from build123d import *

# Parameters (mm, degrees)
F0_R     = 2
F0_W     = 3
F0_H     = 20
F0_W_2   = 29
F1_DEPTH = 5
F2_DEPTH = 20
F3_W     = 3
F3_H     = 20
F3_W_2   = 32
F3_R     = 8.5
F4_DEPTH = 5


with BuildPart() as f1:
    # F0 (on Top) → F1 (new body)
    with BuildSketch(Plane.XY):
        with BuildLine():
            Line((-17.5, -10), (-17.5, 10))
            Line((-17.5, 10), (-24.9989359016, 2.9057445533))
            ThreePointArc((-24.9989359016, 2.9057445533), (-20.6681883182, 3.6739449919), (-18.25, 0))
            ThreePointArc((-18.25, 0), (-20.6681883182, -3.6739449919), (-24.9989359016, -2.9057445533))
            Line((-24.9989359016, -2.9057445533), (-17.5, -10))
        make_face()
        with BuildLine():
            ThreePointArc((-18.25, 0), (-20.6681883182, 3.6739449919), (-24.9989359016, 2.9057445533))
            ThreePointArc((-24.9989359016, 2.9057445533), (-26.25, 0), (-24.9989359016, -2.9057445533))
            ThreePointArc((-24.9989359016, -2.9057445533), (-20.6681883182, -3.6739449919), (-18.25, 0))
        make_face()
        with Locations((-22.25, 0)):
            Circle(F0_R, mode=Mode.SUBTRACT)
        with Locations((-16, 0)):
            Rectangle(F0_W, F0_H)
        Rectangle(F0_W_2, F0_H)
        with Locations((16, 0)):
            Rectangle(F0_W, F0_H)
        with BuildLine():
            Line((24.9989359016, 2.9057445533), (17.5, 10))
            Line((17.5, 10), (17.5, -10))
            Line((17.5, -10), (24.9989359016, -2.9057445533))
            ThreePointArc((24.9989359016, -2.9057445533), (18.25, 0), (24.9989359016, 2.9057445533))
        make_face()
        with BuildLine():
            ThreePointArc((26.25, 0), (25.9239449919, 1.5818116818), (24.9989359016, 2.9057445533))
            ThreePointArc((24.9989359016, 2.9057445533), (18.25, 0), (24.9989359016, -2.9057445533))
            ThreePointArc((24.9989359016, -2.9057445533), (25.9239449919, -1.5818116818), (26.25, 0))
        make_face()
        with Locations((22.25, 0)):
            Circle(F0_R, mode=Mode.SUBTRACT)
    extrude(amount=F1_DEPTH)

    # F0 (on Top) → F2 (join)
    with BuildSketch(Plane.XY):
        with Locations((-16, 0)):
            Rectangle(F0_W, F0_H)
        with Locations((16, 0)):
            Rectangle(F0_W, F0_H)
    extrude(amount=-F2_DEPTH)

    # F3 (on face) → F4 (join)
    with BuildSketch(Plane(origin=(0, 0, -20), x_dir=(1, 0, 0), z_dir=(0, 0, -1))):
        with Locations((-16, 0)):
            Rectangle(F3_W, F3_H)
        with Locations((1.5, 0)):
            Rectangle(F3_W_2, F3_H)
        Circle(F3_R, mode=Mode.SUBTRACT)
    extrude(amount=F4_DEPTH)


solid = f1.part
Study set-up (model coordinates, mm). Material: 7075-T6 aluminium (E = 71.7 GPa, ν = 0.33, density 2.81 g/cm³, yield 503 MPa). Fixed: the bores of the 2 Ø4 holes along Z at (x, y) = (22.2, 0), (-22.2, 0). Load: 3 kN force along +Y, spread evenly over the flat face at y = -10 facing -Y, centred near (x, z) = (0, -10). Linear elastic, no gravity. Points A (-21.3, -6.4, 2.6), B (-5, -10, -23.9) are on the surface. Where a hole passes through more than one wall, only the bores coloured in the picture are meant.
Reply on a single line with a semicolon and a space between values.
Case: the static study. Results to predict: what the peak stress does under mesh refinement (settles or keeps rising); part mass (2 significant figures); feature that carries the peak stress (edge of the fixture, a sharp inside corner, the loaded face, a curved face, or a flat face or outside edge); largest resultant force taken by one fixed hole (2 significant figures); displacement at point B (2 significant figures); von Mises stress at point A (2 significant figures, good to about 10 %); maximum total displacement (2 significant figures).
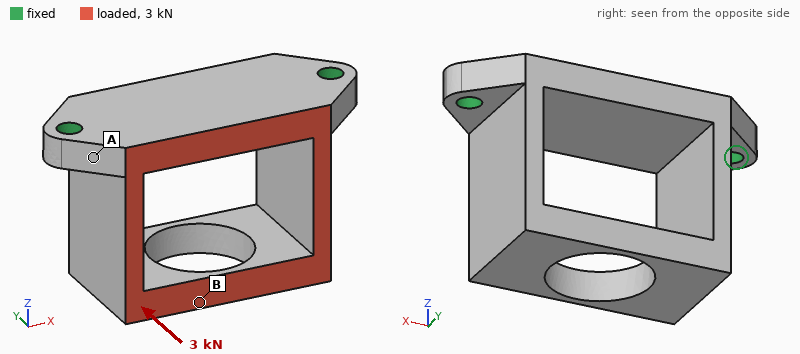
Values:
keeps rising; 26 g; edge of the fixture; 1.5 kN; 0.24 mm; 170 MPa; 0.25 mm
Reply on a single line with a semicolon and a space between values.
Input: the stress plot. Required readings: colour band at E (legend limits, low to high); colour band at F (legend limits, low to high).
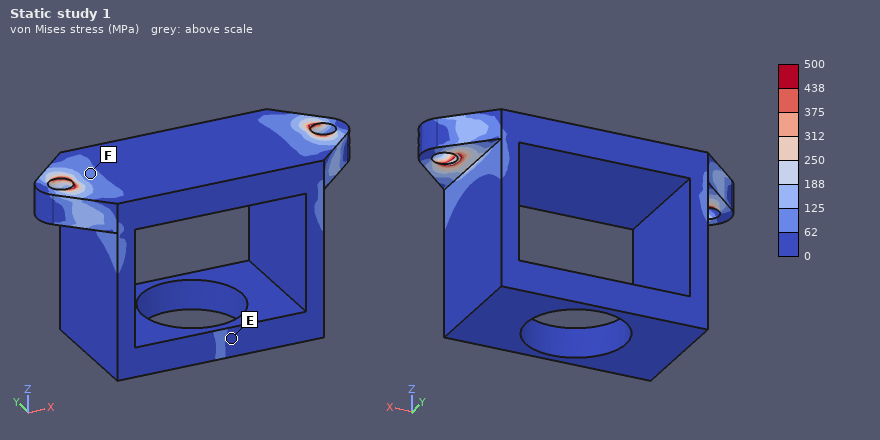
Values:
0 to 62 MPa; 62 to 125 MPa
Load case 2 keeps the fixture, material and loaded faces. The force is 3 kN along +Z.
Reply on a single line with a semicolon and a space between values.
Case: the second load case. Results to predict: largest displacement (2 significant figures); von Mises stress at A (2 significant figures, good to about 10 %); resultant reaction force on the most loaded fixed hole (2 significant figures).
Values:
0.24 mm; 140 MPa; 1.5 kN
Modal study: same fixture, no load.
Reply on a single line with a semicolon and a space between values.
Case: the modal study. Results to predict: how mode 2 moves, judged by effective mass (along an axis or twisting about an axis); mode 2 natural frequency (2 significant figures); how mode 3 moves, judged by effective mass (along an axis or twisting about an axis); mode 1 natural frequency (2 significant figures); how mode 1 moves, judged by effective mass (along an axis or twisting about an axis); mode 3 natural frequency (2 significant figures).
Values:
along Y; 4400 Hz; twisting about Z; 3900 Hz; along X; 7100 Hz
